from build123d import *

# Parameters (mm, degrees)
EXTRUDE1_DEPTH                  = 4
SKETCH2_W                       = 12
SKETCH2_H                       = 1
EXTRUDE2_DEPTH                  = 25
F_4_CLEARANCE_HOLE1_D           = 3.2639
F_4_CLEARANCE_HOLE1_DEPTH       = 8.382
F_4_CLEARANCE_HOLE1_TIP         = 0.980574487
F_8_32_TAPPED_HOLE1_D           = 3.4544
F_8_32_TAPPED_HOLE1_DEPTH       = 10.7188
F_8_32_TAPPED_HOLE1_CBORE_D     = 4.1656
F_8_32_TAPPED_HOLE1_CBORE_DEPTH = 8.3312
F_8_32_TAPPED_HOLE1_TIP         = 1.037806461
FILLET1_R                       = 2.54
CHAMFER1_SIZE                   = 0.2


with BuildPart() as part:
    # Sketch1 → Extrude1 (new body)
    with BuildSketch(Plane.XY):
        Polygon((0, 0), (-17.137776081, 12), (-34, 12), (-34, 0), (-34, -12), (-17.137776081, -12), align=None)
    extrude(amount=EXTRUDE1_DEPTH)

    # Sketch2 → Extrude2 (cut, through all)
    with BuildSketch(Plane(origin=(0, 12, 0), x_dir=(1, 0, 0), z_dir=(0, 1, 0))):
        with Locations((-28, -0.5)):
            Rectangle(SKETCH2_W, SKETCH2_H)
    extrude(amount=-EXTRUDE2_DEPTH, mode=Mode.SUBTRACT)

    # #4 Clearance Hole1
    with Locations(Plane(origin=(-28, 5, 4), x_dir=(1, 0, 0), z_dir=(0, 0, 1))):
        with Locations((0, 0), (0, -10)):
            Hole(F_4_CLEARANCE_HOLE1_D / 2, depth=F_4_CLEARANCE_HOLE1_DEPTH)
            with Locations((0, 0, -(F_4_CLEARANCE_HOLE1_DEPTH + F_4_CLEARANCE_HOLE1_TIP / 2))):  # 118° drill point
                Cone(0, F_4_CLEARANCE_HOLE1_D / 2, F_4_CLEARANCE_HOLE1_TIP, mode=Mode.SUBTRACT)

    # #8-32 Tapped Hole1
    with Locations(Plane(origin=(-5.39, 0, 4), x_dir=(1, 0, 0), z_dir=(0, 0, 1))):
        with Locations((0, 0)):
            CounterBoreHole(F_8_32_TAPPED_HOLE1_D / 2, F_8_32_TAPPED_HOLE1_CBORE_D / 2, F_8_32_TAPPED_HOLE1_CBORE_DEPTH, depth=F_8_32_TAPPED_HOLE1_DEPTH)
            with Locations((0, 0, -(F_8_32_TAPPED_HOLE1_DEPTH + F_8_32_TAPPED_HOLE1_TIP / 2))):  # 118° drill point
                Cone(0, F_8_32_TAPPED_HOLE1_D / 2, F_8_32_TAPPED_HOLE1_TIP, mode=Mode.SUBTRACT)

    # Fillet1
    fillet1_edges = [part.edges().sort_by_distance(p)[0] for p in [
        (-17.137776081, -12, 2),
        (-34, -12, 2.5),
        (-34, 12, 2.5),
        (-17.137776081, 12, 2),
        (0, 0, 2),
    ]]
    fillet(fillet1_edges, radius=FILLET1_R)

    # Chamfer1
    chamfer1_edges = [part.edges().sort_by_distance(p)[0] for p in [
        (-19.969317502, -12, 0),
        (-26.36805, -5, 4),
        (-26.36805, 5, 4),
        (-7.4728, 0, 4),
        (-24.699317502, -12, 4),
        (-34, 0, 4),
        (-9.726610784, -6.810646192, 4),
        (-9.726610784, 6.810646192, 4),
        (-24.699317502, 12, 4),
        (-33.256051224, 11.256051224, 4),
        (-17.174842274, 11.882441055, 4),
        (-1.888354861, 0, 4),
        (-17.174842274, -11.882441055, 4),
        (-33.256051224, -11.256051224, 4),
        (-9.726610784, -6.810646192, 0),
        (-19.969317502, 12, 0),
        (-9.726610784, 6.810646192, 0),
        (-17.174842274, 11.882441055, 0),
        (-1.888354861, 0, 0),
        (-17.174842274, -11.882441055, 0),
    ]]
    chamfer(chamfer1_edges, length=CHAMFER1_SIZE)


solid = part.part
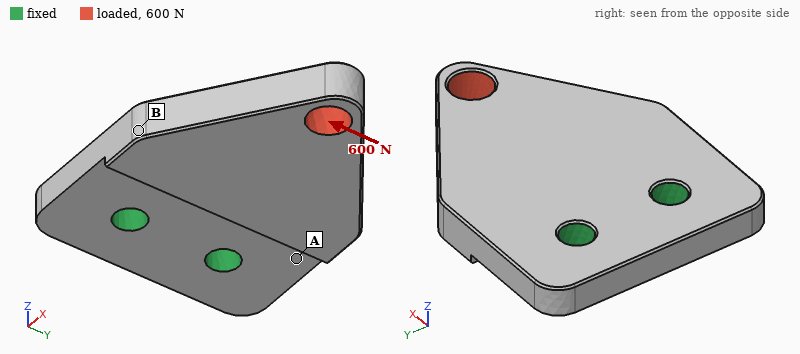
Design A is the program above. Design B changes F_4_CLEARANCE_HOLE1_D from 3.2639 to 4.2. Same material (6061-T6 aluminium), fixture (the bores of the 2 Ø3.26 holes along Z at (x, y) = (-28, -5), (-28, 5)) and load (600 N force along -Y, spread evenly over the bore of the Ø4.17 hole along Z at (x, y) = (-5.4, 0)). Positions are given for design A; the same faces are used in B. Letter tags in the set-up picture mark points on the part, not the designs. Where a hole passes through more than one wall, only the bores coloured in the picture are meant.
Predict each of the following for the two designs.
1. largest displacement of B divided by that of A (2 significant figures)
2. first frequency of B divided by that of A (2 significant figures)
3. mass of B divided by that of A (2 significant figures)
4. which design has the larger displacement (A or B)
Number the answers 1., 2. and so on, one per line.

1. 0.91
2. 1.1
3. 0.98
4. A
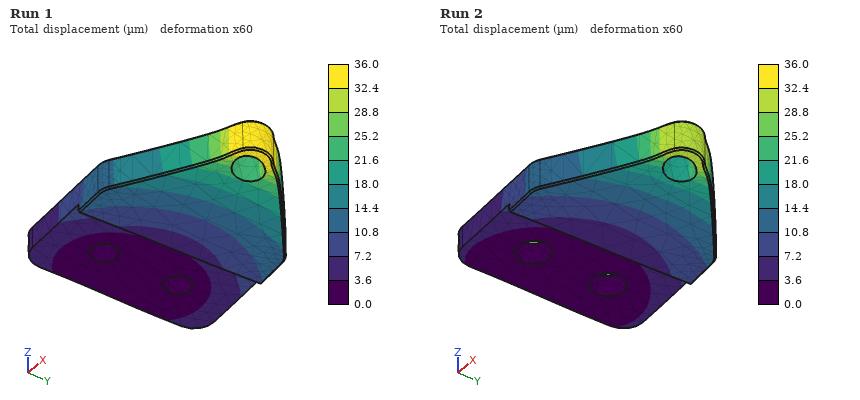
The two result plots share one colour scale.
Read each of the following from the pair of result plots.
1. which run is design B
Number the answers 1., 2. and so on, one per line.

1. Run 2
